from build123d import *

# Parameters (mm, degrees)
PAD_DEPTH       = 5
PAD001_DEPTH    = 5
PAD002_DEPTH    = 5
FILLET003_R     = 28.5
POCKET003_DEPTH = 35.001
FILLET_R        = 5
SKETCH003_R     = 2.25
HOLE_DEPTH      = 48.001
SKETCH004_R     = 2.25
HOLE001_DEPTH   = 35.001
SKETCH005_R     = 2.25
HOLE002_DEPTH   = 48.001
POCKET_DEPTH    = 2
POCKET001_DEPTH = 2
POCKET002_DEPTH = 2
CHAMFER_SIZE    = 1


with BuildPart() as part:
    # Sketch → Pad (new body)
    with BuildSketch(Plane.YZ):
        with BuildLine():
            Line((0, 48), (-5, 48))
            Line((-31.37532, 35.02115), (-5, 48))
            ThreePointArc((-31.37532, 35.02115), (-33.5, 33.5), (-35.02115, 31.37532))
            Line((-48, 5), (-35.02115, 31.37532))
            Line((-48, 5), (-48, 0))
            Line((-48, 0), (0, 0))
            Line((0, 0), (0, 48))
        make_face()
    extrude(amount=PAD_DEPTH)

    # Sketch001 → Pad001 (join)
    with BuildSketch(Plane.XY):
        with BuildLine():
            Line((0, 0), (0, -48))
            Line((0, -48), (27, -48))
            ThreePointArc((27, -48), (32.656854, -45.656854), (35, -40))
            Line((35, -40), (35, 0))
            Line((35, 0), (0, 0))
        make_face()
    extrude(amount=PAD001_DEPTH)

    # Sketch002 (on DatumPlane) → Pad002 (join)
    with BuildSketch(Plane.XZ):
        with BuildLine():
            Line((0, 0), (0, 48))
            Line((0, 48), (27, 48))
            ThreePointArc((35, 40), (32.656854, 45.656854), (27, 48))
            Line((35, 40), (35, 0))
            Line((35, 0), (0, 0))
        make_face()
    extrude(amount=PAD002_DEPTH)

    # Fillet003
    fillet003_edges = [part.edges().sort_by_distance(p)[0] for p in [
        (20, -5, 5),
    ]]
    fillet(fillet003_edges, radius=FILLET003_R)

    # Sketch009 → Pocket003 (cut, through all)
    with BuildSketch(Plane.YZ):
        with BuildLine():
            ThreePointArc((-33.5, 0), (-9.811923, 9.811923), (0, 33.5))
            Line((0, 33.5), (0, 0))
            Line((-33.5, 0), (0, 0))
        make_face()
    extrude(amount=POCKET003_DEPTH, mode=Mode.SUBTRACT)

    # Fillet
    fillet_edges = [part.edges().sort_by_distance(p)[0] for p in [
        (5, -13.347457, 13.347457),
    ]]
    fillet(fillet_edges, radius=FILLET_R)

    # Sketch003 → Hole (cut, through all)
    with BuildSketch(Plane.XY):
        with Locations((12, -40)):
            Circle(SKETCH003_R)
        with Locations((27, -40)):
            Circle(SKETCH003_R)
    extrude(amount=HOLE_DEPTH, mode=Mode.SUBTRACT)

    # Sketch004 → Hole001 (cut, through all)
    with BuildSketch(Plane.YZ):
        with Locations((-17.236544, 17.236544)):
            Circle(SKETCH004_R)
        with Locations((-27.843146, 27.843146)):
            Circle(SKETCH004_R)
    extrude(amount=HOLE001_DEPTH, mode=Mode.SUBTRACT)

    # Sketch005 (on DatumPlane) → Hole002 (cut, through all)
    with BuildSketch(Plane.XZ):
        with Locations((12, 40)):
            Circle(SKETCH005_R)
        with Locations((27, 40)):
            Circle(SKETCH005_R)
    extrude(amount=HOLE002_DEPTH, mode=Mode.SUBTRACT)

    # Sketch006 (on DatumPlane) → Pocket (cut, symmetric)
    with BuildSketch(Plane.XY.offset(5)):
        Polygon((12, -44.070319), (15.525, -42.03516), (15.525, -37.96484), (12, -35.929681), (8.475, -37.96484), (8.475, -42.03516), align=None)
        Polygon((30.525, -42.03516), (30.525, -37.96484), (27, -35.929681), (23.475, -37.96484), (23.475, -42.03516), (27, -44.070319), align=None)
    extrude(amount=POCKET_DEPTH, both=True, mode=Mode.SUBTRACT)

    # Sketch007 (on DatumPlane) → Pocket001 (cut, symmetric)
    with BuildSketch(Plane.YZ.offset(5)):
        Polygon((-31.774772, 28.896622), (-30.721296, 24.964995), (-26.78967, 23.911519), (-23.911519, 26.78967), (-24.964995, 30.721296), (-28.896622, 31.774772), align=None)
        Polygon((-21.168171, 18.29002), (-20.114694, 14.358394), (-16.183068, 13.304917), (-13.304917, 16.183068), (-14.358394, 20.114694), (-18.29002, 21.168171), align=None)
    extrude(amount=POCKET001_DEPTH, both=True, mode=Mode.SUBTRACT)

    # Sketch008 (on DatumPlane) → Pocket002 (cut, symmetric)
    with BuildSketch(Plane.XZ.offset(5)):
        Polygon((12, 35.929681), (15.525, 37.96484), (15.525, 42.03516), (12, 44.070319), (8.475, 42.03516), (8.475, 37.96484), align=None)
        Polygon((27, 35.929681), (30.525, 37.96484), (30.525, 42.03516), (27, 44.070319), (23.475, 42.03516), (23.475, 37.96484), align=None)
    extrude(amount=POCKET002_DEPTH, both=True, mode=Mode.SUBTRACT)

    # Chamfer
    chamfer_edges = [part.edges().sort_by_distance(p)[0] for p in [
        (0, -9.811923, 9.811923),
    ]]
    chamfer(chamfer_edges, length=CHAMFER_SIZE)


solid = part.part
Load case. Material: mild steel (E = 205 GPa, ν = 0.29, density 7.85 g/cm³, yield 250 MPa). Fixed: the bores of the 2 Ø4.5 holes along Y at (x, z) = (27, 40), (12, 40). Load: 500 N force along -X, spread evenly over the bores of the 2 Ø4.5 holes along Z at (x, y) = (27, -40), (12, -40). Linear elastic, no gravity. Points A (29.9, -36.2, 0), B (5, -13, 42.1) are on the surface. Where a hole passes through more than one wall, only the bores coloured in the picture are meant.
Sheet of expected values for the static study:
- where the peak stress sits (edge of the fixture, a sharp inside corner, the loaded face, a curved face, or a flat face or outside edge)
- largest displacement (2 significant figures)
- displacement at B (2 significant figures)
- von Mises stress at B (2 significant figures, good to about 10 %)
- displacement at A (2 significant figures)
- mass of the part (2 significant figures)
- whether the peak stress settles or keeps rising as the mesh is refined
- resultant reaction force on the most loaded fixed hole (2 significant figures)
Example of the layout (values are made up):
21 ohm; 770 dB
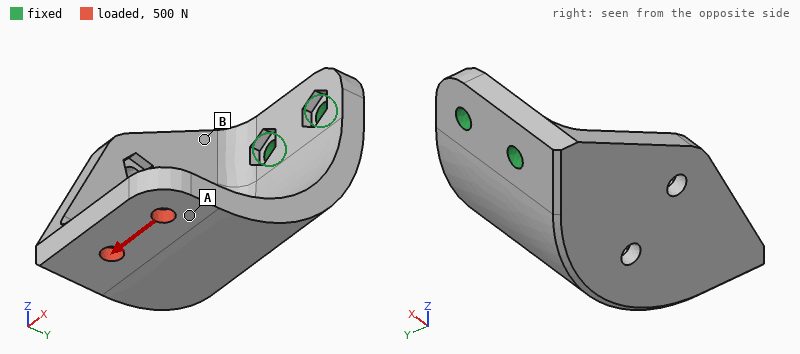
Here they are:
edge of the fixture; 0.11 mm; 0.018 mm; 30 MPa; 0.069 mm; 140 g; keeps rising; 1.6 kN
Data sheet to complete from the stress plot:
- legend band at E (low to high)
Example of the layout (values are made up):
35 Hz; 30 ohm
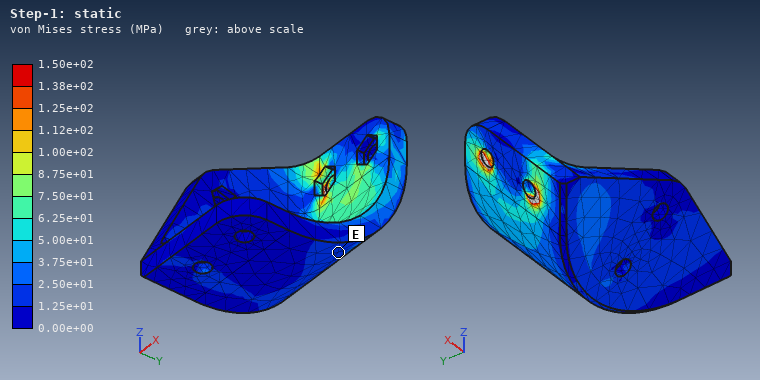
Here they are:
1.25e+01 to 2.50e+01 MPa
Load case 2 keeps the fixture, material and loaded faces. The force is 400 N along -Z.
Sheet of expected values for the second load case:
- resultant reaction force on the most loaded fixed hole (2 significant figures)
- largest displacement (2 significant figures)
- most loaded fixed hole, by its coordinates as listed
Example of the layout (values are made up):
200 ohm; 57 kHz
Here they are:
310 N; 0.16 mm; (27, 40)
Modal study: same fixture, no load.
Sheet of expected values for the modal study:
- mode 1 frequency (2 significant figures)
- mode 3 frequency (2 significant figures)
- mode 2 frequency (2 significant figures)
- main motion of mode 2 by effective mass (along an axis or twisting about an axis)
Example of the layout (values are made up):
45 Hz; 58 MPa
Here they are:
1100 Hz; 5200 Hz; 1800 Hz; along X
